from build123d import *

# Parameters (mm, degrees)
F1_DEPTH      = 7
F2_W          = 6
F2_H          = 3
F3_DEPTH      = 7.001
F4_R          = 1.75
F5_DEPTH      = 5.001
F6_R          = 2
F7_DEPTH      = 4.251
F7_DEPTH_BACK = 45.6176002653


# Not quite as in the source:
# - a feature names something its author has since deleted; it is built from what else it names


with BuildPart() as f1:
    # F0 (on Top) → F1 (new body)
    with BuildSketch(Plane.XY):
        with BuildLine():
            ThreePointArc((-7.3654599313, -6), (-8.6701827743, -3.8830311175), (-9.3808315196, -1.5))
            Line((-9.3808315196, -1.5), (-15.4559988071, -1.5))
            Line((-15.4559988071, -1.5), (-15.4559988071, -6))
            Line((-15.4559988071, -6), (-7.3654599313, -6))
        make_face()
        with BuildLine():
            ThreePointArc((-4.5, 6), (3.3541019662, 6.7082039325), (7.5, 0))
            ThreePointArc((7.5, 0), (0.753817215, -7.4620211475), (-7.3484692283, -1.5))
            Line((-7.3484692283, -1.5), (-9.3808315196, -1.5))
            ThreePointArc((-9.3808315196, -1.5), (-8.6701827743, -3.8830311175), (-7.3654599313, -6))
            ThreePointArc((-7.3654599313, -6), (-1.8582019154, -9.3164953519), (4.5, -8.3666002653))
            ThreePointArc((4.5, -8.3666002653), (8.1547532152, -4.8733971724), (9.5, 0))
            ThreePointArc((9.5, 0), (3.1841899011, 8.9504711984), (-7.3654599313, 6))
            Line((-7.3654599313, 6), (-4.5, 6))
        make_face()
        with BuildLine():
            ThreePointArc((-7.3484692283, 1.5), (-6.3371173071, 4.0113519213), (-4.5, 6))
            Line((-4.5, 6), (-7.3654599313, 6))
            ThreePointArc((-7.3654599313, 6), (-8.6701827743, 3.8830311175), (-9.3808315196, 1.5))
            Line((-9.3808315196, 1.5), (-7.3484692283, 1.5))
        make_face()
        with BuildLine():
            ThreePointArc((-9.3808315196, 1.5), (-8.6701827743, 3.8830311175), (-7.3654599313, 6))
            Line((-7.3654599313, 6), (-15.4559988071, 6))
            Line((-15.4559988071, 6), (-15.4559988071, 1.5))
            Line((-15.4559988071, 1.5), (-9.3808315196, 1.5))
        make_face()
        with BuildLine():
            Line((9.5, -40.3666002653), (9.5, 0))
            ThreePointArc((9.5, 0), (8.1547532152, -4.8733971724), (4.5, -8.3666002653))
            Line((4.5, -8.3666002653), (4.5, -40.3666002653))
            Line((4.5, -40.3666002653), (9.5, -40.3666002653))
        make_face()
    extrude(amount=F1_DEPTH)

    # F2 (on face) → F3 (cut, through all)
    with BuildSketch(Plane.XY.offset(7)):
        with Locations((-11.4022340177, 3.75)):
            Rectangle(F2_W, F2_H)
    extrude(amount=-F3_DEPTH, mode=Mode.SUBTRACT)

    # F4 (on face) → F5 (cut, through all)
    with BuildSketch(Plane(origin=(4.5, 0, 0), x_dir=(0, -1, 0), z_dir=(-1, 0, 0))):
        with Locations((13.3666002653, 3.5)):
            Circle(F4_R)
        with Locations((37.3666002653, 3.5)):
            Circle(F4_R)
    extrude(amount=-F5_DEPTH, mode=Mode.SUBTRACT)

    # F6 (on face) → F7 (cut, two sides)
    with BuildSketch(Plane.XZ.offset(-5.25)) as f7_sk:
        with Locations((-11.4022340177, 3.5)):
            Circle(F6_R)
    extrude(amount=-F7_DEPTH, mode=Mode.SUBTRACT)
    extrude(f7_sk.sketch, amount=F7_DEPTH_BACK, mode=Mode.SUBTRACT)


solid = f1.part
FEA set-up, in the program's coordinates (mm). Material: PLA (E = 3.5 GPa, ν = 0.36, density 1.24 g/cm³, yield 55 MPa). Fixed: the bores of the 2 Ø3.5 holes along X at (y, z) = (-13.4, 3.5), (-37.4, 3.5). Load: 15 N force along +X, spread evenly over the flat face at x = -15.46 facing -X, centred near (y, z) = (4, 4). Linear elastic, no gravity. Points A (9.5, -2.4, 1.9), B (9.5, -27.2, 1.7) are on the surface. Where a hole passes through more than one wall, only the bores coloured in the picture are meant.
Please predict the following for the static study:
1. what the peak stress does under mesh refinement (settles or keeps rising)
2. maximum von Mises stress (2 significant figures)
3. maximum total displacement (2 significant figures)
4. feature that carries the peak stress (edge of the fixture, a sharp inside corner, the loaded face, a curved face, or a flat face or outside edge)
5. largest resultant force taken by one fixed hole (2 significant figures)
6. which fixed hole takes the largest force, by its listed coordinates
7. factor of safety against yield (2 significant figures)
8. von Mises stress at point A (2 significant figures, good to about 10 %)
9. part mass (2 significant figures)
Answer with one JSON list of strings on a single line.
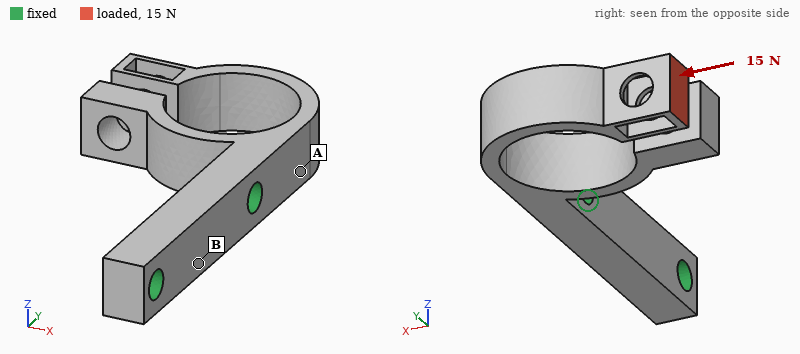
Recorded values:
["settles", "18 MPa", "0.49 mm", "a curved face", "15 N", "(-13.4, 3.5)", "3.1", "13 MPa", "2.5 g"]
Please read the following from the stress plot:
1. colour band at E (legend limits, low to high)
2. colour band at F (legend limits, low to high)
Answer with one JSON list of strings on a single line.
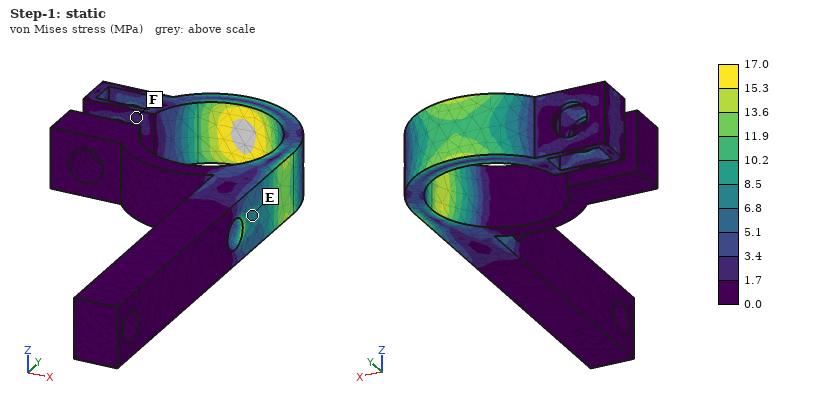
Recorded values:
["6.8 to 8.5 MPa", "1.7 to 3.4 MPa"]
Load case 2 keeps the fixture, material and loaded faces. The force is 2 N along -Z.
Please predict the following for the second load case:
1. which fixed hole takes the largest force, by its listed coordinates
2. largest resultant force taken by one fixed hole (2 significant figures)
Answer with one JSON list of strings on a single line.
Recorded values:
["(-13.4, 3.5)", "2.2 N"]
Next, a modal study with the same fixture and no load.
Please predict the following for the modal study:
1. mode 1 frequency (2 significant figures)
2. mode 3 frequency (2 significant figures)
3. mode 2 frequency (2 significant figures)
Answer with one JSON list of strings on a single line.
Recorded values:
["580 Hz", "890 Hz", "760 Hz"]
